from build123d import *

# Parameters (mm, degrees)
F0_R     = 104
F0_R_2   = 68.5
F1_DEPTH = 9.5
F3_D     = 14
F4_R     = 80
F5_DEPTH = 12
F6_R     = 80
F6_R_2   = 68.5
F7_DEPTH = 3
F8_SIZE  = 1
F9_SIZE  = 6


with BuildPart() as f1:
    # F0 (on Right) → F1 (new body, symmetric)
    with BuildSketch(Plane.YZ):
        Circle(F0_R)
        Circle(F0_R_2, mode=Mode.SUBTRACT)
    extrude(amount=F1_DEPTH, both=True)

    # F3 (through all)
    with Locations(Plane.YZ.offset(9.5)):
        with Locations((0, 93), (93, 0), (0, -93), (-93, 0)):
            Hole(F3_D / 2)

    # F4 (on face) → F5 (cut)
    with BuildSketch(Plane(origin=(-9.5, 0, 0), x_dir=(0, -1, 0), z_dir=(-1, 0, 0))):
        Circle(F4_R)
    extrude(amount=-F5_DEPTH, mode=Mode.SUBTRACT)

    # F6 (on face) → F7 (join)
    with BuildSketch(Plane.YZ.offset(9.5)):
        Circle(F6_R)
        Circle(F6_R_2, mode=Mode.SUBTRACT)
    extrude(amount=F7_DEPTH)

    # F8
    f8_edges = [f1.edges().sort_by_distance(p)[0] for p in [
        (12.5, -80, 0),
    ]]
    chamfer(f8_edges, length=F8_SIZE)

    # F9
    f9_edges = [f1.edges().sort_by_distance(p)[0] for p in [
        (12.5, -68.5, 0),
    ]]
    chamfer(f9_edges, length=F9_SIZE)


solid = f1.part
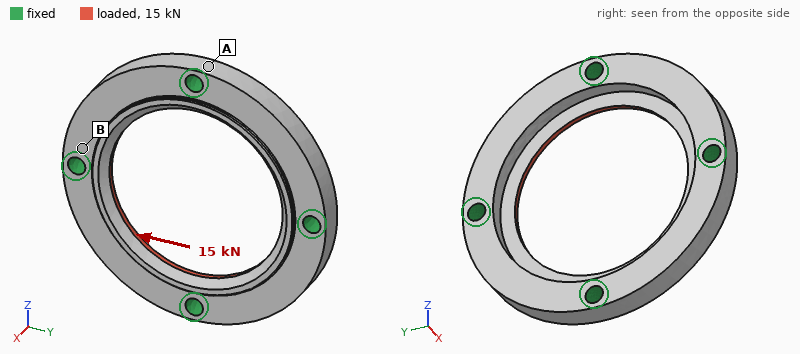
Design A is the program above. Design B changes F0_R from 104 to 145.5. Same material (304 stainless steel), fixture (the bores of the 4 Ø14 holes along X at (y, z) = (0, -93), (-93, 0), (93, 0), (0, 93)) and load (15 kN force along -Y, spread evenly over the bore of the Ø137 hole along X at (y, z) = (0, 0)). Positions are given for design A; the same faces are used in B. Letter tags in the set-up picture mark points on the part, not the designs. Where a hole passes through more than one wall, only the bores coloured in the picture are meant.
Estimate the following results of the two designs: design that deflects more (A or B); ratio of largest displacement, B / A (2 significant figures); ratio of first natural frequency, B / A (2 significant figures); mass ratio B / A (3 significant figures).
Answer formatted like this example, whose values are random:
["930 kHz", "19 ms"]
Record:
["A", "0.62", "0.44", "3.08"]
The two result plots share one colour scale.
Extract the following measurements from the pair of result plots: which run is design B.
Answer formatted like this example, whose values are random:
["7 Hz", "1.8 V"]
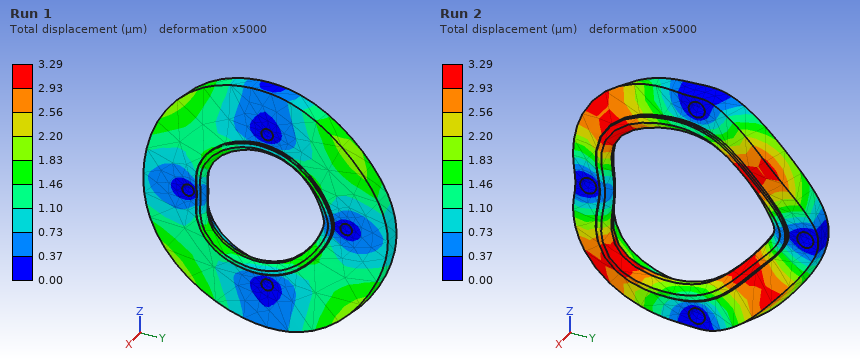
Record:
["Run 1"]
